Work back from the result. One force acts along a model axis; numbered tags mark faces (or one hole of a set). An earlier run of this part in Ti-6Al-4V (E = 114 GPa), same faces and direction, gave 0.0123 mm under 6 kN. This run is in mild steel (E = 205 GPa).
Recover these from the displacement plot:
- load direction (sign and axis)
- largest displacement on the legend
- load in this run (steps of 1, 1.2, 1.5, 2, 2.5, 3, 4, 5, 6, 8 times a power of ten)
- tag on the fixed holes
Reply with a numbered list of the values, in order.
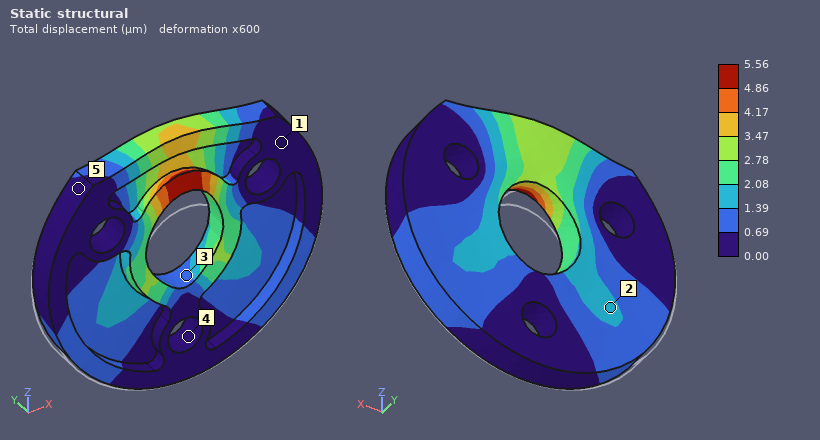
1. +Z
2. 5.56 µm
3. 5 kN
4. 4
